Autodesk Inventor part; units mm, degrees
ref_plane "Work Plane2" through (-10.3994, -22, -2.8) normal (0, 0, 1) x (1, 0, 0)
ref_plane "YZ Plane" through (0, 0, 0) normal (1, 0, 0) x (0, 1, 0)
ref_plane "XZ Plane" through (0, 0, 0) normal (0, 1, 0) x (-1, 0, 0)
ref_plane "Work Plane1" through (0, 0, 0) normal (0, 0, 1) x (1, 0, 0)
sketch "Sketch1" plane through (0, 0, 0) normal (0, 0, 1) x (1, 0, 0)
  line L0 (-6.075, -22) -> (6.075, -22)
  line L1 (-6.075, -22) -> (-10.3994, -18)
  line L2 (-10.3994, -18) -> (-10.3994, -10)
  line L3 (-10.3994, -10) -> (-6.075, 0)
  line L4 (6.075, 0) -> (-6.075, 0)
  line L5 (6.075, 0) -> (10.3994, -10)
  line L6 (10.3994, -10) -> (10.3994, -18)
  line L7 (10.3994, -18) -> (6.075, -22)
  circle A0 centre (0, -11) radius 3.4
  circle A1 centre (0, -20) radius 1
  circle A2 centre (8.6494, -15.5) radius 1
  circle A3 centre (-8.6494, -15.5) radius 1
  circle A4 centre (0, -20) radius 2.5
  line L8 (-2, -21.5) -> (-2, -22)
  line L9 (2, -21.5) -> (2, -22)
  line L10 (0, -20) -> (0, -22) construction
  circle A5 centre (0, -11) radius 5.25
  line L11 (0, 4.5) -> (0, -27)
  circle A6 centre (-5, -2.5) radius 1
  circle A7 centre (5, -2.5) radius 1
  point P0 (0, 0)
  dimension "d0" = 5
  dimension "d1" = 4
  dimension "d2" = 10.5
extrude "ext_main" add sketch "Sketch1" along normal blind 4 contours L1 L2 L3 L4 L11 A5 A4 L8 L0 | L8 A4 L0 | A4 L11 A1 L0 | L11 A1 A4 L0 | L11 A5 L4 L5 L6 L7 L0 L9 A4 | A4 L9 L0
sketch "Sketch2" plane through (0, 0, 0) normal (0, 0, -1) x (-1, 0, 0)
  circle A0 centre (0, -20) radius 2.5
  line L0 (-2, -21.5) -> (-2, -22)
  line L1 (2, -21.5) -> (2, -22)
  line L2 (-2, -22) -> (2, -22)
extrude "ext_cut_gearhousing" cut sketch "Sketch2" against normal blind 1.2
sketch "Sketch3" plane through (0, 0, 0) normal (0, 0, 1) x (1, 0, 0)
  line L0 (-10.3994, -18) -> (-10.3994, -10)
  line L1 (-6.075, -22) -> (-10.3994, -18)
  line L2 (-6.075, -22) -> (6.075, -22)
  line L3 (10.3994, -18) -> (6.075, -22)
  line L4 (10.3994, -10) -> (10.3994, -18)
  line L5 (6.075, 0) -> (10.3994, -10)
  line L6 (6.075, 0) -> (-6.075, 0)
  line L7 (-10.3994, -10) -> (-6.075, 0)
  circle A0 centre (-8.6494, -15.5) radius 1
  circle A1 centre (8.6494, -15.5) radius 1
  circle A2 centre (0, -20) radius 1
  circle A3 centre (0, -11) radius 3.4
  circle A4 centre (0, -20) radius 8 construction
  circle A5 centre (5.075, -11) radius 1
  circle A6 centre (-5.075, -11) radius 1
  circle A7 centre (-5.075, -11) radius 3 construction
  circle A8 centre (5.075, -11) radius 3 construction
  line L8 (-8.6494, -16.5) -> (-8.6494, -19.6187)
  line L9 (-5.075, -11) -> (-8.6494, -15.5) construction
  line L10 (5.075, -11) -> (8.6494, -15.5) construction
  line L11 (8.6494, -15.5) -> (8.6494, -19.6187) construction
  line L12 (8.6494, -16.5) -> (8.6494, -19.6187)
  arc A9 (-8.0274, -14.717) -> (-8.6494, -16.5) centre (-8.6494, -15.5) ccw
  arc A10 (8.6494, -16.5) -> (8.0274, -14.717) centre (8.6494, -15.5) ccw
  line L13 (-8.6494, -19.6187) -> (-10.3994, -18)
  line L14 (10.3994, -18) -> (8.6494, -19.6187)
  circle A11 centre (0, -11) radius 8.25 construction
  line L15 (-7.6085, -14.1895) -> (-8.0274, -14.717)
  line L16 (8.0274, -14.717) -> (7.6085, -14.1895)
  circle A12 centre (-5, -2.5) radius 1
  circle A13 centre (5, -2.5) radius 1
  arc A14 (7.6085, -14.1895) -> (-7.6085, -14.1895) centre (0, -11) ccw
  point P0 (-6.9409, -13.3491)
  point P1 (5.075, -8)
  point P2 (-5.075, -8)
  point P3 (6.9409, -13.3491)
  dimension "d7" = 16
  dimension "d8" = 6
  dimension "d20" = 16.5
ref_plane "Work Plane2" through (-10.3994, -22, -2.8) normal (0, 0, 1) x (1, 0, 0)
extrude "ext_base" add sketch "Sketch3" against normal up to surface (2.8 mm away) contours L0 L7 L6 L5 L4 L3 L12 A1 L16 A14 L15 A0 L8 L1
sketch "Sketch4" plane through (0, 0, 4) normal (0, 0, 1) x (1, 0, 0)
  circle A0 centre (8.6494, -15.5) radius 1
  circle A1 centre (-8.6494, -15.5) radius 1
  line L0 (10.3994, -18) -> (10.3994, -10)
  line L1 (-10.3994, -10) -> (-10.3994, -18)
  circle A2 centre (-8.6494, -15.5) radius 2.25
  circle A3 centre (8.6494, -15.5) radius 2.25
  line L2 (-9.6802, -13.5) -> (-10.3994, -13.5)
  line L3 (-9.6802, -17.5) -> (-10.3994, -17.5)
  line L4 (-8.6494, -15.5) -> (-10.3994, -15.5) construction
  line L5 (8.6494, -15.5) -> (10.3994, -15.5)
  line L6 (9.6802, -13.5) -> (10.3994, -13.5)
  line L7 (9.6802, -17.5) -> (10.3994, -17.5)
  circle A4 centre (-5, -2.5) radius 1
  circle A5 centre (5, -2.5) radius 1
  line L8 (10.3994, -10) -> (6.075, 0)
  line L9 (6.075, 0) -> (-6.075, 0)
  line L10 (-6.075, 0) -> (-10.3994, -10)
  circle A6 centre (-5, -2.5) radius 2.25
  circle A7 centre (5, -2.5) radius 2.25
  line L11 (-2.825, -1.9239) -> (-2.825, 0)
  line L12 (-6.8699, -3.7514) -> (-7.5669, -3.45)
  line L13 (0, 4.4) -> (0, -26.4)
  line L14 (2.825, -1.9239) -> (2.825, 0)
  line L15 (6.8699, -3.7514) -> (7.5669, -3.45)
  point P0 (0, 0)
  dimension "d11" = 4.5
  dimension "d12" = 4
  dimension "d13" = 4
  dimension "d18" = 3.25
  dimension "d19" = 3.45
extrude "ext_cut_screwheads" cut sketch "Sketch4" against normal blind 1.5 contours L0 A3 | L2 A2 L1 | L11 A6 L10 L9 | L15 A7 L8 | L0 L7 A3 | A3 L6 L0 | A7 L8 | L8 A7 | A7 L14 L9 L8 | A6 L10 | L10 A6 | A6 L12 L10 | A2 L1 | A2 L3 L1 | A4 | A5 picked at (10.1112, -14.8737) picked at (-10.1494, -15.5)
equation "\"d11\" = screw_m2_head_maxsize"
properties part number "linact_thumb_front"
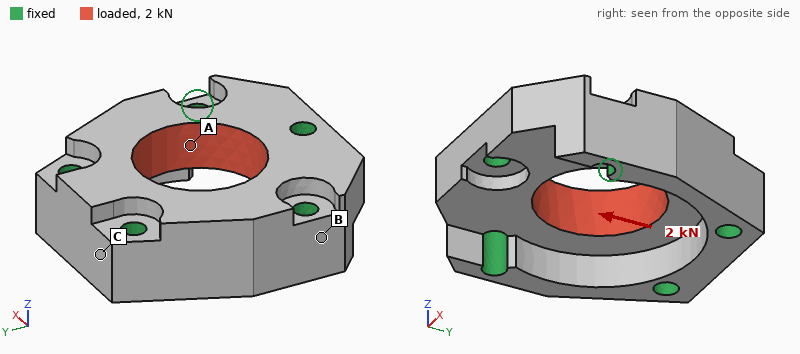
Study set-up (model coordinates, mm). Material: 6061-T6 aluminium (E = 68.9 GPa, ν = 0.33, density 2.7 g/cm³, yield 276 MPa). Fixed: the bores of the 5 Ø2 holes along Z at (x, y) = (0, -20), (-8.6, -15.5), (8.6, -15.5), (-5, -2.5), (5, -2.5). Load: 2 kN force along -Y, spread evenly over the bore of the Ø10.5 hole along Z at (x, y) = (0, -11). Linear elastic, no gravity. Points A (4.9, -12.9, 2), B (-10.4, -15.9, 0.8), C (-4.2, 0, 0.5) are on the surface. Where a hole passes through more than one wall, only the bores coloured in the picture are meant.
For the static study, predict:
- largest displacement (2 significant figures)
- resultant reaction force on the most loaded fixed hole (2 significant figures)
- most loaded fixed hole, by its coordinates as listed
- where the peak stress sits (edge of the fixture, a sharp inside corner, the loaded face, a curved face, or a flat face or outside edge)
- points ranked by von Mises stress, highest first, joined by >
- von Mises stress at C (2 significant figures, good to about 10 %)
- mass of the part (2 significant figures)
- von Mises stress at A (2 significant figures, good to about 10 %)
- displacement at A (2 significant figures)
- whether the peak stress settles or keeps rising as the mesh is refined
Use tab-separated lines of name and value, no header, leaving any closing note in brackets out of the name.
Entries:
largest displacement	3.4 µm
resultant reaction force on the most loaded fixed hole	500 N
most loaded fixed hole, by its coordinates as listed	(0, -20)
where the peak stress sits	edge of the fixture
points ranked by von Mises stress, highest first, joined by >	A > C > B
von Mises stress at C	12 MPa
mass of the part	3.7 g
von Mises stress at A	26 MPa
displacement at A	2.1 µm
whether the peak stress settles or keeps rising as the mesh is refined	keeps rising
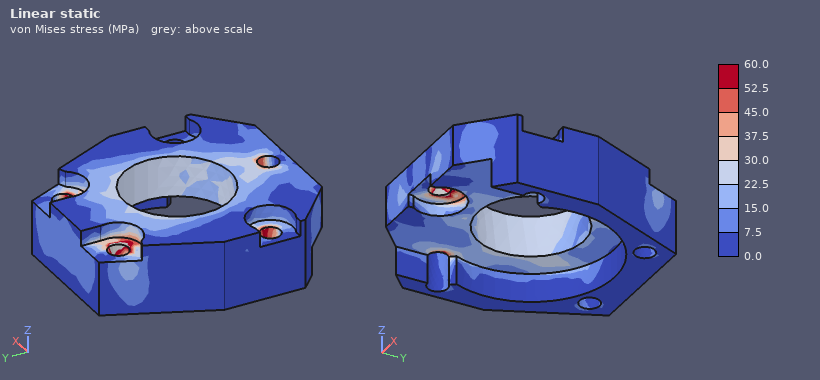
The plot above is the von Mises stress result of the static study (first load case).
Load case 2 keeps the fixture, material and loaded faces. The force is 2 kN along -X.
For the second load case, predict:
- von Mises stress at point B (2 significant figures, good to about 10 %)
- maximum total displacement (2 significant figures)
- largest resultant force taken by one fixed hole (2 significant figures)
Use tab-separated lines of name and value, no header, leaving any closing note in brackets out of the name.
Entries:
von Mises stress at point B	13 MPa
maximum total displacement	5.0 µm
largest resultant force taken by one fixed hole	430 N
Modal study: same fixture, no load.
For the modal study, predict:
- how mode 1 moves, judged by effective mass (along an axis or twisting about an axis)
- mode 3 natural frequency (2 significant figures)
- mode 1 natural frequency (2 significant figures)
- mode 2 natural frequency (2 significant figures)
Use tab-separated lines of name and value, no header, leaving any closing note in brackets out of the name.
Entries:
how mode 1 moves, judged by effective mass	along Z
mode 3 natural frequency	87 kHz
mode 1 natural frequency	82 kHz
mode 2 natural frequency	85 kHz
